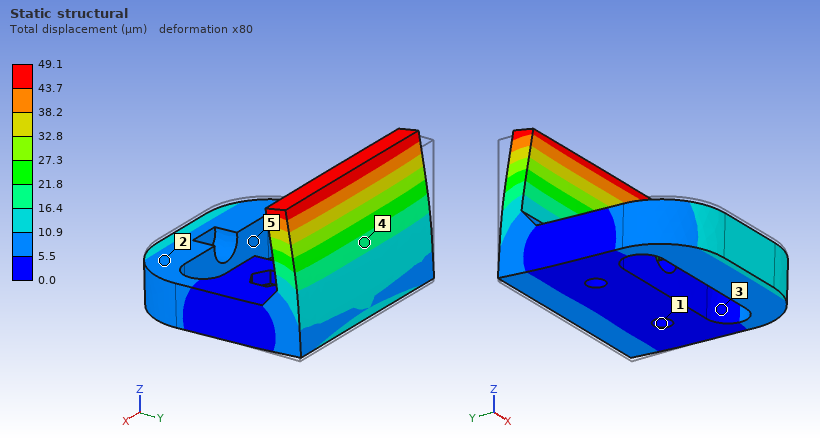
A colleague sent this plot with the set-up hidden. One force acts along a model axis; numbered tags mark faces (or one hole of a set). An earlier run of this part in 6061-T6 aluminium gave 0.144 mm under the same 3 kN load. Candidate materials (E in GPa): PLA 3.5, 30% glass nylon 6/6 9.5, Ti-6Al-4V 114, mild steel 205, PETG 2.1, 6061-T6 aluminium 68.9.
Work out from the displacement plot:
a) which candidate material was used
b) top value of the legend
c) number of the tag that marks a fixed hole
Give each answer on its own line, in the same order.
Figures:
mild steel
49.1 µm
1
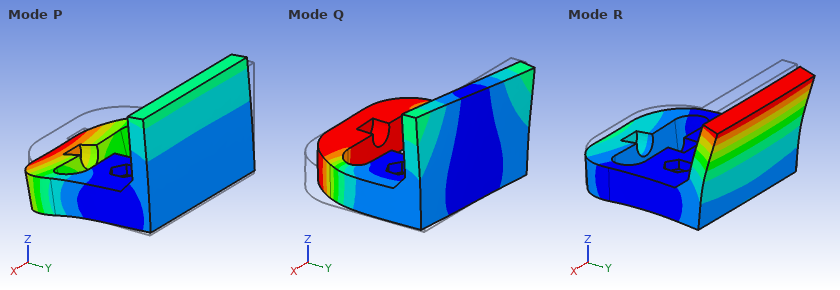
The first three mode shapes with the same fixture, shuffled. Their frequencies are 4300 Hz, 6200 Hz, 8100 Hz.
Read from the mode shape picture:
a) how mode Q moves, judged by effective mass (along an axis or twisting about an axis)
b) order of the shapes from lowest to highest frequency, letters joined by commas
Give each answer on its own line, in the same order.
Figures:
along X
P, R, Q
